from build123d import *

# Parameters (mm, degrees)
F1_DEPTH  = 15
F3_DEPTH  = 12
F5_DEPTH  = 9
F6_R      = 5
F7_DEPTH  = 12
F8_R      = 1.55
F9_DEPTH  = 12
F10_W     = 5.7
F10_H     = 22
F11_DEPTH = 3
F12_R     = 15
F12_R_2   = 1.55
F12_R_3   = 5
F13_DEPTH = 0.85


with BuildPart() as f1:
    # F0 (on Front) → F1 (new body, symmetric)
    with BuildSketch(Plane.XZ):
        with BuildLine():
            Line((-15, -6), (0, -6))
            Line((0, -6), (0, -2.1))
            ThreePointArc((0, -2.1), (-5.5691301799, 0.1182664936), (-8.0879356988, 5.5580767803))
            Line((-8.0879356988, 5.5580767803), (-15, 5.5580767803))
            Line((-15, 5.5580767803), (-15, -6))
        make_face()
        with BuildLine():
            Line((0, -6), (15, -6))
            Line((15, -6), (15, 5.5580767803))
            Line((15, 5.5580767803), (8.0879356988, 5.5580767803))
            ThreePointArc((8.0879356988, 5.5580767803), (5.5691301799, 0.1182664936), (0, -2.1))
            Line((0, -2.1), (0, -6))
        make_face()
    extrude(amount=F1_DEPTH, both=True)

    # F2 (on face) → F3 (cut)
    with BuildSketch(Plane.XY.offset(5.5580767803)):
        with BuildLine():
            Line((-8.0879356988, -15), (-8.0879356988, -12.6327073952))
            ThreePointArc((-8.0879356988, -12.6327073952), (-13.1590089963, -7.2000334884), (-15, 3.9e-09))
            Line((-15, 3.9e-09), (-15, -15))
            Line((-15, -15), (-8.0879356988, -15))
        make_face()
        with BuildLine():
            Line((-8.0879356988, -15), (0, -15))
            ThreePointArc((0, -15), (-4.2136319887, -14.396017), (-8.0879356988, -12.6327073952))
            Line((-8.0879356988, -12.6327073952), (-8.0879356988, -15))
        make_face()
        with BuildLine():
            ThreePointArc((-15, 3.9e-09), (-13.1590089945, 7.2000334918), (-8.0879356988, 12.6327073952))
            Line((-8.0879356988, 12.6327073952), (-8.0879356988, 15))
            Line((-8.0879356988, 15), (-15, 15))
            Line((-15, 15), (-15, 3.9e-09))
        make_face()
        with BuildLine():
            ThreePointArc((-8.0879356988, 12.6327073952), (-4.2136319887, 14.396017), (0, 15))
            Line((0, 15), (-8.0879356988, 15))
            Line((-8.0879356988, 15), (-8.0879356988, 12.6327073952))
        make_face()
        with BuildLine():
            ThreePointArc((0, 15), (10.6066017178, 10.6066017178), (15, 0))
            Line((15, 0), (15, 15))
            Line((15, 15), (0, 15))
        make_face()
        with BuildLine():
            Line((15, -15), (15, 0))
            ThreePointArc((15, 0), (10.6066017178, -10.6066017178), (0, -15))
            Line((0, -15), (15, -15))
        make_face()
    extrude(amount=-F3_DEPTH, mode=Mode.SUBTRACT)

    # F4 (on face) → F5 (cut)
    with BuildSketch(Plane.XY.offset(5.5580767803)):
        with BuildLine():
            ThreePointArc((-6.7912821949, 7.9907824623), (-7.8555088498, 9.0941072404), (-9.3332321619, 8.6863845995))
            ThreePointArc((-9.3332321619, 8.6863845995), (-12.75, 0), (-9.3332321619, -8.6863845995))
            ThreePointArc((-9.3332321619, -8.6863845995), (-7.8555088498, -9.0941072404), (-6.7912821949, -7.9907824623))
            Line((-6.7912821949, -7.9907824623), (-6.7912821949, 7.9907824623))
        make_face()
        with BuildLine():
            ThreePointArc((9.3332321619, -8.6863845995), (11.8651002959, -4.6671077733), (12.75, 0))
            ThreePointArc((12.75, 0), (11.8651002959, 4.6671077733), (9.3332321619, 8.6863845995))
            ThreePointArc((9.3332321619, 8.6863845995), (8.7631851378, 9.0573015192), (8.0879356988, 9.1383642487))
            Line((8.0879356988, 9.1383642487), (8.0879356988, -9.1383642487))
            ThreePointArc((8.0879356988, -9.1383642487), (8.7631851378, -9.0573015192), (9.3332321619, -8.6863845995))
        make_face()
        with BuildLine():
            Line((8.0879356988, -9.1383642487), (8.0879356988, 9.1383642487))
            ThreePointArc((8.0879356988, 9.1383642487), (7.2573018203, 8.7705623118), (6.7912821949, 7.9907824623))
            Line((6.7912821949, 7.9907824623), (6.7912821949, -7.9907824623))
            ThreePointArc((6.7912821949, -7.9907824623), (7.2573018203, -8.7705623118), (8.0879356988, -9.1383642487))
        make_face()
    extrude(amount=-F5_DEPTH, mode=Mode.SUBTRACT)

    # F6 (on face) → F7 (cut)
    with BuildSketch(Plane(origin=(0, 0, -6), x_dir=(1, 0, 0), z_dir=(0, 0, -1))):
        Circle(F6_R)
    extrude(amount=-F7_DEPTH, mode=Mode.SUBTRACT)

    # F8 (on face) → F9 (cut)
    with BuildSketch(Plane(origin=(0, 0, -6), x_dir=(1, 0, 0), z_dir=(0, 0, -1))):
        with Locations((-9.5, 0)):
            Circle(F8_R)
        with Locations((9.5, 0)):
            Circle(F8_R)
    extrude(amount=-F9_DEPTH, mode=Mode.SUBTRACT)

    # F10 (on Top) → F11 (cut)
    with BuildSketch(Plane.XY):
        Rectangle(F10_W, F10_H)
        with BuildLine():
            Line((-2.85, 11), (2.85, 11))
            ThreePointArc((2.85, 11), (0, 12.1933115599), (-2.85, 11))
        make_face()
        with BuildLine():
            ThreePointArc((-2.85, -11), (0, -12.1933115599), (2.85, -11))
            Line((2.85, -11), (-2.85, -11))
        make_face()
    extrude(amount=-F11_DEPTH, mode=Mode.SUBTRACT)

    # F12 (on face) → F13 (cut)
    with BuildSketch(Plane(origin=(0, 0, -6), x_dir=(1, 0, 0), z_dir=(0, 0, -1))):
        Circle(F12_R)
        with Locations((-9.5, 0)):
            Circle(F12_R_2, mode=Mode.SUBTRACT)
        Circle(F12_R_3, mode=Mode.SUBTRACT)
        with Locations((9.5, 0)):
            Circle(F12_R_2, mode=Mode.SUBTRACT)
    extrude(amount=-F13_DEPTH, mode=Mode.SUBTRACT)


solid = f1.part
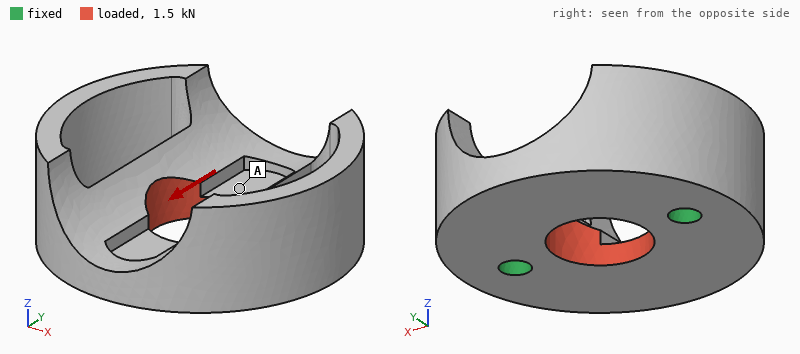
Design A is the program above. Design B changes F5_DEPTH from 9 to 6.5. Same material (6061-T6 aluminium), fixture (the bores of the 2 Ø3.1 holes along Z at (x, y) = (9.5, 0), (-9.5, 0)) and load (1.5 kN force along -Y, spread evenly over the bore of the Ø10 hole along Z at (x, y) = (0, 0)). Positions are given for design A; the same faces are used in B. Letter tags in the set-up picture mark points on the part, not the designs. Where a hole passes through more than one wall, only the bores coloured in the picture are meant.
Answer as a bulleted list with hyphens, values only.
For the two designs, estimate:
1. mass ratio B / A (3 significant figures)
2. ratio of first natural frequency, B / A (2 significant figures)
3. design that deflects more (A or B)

- 1.13
- 2.4
- A
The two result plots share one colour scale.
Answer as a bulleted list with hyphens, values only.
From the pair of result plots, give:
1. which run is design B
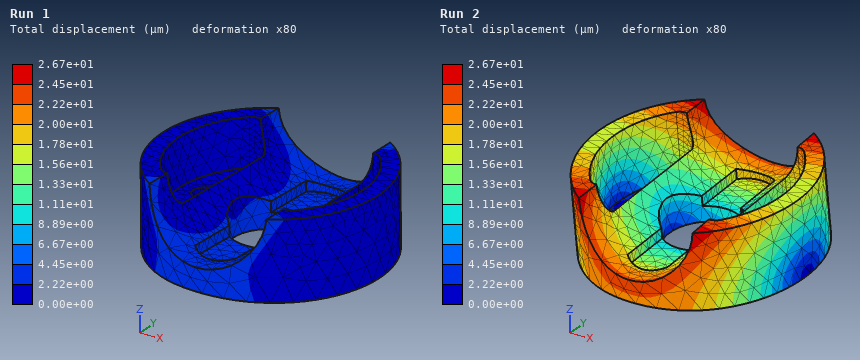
- Run 1
